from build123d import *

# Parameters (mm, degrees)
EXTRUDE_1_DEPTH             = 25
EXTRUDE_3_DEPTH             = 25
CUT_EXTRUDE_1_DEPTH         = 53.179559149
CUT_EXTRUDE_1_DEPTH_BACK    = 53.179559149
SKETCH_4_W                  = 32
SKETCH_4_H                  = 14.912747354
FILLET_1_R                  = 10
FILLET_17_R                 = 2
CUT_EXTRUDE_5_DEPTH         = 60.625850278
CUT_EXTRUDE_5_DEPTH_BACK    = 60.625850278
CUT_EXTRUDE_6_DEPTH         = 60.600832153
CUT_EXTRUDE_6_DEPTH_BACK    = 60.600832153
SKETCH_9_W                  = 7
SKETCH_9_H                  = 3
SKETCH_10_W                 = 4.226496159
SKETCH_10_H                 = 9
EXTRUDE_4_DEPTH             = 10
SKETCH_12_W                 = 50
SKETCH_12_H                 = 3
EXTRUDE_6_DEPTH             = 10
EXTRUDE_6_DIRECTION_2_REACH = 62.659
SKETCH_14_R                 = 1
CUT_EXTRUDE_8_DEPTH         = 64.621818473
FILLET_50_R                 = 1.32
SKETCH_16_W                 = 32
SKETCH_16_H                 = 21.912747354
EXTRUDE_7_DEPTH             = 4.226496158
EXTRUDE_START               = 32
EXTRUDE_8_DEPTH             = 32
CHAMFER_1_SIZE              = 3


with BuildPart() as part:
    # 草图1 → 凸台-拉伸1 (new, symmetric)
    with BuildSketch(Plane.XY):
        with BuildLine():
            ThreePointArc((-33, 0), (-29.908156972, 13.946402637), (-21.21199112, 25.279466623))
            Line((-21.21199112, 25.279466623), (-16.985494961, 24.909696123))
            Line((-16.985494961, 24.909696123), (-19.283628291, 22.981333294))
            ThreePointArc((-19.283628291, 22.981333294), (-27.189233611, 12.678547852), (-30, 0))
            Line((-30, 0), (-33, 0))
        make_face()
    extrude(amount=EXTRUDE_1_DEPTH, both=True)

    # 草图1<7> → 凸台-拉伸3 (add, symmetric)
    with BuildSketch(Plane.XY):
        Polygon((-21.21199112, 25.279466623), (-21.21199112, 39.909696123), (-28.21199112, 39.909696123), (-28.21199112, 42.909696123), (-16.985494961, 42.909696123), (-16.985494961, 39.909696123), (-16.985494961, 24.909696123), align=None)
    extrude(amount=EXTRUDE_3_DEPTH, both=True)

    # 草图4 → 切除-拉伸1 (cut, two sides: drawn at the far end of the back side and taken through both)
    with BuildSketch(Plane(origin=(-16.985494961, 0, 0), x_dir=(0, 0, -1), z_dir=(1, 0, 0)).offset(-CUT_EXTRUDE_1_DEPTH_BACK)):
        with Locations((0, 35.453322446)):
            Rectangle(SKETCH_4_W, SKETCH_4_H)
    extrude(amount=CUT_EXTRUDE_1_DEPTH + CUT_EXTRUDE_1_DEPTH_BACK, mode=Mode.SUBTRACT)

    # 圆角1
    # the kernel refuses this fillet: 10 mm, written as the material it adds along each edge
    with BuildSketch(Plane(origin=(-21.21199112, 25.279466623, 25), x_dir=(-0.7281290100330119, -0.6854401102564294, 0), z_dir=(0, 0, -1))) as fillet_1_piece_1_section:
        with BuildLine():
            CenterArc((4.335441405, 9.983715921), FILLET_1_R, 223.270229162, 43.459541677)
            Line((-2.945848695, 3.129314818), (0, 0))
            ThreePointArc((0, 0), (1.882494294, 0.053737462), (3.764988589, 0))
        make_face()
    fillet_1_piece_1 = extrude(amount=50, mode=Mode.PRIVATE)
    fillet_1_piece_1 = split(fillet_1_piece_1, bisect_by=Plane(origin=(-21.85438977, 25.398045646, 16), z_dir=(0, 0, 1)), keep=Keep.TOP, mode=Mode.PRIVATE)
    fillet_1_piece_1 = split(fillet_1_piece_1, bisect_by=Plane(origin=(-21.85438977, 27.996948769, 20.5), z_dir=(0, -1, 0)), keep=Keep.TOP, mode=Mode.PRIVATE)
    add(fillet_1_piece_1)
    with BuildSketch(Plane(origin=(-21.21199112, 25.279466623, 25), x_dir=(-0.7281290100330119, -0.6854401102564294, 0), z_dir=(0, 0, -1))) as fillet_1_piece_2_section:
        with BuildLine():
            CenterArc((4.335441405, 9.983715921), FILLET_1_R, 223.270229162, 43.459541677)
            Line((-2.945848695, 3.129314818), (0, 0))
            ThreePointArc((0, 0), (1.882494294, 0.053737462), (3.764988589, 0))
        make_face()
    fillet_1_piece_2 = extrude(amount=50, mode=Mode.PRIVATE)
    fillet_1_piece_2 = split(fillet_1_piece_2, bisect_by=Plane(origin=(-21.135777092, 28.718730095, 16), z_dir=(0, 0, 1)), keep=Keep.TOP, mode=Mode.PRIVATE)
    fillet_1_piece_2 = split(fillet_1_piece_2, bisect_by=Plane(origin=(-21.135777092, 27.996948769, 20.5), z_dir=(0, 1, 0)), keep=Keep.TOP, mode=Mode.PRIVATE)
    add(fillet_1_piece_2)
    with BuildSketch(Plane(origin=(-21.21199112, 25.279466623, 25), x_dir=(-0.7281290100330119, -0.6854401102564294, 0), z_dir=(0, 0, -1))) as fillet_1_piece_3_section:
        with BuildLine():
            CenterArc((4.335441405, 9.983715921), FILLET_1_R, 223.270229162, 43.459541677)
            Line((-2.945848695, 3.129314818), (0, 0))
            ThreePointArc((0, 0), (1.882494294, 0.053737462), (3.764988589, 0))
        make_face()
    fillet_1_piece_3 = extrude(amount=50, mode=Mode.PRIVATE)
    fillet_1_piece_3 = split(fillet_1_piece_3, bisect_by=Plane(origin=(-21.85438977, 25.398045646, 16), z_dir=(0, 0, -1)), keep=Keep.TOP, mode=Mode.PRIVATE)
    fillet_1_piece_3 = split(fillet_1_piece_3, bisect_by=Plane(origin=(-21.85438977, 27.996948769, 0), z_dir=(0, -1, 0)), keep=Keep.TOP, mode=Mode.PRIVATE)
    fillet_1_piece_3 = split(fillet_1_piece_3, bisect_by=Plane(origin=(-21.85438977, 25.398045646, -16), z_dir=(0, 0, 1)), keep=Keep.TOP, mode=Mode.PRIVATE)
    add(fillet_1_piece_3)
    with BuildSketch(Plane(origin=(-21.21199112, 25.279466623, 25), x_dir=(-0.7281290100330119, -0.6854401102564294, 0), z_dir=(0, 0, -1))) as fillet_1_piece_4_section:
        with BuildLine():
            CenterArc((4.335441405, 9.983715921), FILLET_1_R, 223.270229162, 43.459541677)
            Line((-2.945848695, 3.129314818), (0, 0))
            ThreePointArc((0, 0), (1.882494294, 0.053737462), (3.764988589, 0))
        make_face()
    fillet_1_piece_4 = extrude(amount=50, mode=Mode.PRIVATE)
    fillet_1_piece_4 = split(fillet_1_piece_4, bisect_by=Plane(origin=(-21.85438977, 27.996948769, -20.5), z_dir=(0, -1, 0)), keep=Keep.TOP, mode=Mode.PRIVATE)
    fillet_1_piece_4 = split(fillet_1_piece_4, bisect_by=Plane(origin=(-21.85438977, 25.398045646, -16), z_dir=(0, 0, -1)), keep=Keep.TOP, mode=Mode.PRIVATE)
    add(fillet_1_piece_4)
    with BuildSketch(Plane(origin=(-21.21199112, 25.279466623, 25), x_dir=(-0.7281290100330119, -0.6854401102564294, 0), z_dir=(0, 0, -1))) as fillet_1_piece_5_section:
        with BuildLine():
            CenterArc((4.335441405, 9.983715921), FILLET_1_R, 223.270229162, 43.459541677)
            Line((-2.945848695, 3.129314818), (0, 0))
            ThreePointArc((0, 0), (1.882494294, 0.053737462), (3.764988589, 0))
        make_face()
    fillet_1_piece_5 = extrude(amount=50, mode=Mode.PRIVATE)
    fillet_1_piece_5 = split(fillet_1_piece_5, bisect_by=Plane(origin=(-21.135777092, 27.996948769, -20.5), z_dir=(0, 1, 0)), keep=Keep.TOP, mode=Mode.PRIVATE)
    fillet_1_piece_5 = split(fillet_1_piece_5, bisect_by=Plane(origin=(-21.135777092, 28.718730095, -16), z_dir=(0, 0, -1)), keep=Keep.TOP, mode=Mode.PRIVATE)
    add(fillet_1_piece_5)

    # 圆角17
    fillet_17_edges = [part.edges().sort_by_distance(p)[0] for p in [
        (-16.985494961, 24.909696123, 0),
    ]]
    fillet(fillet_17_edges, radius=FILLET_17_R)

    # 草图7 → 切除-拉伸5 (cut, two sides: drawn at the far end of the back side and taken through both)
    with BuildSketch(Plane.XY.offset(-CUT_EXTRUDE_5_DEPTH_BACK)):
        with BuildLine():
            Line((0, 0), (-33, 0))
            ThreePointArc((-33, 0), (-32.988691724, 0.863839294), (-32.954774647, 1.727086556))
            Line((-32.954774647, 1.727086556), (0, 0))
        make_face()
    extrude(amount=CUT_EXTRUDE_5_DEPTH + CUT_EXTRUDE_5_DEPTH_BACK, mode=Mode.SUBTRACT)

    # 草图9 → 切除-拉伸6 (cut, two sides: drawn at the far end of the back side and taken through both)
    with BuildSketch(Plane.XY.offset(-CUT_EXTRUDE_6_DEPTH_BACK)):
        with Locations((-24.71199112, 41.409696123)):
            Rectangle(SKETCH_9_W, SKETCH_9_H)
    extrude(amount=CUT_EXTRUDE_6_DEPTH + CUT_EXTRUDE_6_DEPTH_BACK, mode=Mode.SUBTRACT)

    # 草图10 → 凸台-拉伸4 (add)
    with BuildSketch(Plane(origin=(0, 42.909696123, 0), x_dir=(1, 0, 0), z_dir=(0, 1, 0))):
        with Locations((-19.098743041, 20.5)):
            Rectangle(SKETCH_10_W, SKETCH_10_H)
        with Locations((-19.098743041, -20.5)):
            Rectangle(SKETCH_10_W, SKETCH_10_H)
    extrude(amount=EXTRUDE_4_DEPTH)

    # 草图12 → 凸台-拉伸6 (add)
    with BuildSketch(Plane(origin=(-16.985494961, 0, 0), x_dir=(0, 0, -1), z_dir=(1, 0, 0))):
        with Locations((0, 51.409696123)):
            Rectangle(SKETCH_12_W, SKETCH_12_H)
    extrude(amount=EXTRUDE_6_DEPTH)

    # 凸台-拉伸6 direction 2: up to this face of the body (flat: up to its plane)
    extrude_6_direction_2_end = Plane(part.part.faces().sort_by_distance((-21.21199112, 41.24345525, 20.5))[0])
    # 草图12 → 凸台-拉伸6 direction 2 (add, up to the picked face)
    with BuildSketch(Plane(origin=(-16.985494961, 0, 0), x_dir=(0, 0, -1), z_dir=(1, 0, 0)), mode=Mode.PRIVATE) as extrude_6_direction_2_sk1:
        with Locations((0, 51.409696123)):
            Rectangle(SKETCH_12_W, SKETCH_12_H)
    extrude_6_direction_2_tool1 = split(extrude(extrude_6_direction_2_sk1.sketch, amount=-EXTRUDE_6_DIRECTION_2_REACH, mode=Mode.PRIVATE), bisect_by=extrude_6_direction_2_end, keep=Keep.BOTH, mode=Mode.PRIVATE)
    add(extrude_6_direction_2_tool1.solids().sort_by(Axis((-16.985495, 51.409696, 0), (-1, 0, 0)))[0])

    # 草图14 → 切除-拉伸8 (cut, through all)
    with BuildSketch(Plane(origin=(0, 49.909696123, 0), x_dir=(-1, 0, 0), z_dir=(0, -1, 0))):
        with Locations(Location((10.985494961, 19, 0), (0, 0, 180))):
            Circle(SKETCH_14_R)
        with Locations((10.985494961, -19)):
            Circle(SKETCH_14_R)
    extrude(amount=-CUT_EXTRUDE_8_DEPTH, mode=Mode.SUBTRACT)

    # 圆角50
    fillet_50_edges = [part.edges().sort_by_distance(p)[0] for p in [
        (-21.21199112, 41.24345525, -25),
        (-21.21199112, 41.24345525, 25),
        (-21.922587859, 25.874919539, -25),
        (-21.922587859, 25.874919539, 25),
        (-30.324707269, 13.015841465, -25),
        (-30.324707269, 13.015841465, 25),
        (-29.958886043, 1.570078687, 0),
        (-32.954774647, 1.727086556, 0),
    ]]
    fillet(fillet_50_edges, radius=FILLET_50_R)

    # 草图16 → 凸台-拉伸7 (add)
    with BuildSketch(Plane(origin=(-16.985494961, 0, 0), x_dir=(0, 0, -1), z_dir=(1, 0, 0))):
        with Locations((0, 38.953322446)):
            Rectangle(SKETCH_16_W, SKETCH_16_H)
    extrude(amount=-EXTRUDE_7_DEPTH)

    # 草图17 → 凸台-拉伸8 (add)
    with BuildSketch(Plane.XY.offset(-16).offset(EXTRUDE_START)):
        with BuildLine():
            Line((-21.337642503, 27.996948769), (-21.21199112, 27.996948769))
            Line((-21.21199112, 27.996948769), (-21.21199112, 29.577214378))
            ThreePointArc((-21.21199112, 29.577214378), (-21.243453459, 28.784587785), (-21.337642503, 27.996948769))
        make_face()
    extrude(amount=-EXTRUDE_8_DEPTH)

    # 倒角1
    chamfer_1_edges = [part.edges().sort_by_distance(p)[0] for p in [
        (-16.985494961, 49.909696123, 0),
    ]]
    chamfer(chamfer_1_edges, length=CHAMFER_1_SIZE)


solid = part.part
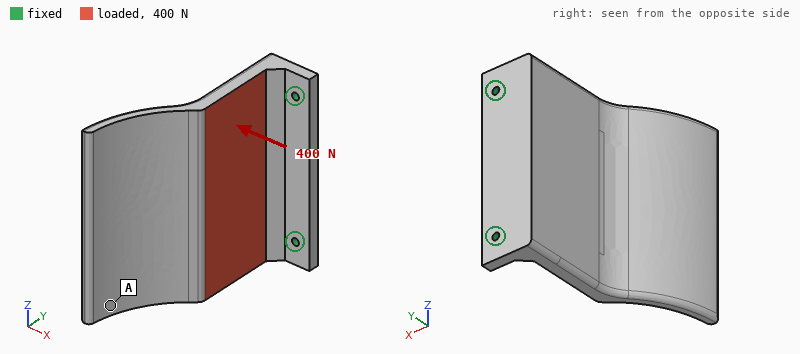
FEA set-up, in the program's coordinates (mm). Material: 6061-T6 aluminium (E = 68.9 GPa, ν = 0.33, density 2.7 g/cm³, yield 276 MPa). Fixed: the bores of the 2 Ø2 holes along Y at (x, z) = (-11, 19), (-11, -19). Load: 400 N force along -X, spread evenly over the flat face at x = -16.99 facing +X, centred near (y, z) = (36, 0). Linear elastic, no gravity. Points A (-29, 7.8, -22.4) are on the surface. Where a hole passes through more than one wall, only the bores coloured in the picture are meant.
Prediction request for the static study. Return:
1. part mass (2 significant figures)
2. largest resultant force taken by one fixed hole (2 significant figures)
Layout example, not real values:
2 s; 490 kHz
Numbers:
32 g; 220 N
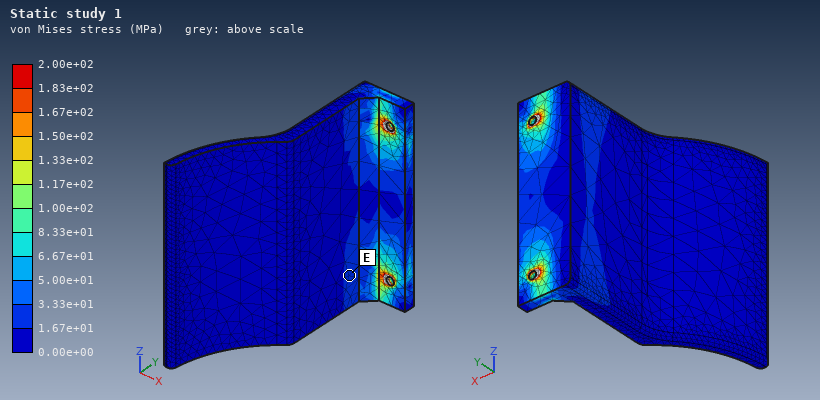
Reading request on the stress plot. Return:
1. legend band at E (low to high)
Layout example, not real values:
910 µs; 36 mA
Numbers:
1.67e+01 to 3.33e+01 MPa
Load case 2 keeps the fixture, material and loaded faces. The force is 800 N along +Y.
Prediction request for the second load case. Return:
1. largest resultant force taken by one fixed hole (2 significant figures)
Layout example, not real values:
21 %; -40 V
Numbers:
400 N
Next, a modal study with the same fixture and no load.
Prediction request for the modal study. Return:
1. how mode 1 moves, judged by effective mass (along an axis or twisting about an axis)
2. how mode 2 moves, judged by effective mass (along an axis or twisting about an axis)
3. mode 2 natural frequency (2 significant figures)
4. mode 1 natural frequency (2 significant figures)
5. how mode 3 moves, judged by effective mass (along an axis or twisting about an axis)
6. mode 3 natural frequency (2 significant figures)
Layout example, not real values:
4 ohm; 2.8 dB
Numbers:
along X; twisting about Y; 2800 Hz; 830 Hz; along Z; 4700 Hz
